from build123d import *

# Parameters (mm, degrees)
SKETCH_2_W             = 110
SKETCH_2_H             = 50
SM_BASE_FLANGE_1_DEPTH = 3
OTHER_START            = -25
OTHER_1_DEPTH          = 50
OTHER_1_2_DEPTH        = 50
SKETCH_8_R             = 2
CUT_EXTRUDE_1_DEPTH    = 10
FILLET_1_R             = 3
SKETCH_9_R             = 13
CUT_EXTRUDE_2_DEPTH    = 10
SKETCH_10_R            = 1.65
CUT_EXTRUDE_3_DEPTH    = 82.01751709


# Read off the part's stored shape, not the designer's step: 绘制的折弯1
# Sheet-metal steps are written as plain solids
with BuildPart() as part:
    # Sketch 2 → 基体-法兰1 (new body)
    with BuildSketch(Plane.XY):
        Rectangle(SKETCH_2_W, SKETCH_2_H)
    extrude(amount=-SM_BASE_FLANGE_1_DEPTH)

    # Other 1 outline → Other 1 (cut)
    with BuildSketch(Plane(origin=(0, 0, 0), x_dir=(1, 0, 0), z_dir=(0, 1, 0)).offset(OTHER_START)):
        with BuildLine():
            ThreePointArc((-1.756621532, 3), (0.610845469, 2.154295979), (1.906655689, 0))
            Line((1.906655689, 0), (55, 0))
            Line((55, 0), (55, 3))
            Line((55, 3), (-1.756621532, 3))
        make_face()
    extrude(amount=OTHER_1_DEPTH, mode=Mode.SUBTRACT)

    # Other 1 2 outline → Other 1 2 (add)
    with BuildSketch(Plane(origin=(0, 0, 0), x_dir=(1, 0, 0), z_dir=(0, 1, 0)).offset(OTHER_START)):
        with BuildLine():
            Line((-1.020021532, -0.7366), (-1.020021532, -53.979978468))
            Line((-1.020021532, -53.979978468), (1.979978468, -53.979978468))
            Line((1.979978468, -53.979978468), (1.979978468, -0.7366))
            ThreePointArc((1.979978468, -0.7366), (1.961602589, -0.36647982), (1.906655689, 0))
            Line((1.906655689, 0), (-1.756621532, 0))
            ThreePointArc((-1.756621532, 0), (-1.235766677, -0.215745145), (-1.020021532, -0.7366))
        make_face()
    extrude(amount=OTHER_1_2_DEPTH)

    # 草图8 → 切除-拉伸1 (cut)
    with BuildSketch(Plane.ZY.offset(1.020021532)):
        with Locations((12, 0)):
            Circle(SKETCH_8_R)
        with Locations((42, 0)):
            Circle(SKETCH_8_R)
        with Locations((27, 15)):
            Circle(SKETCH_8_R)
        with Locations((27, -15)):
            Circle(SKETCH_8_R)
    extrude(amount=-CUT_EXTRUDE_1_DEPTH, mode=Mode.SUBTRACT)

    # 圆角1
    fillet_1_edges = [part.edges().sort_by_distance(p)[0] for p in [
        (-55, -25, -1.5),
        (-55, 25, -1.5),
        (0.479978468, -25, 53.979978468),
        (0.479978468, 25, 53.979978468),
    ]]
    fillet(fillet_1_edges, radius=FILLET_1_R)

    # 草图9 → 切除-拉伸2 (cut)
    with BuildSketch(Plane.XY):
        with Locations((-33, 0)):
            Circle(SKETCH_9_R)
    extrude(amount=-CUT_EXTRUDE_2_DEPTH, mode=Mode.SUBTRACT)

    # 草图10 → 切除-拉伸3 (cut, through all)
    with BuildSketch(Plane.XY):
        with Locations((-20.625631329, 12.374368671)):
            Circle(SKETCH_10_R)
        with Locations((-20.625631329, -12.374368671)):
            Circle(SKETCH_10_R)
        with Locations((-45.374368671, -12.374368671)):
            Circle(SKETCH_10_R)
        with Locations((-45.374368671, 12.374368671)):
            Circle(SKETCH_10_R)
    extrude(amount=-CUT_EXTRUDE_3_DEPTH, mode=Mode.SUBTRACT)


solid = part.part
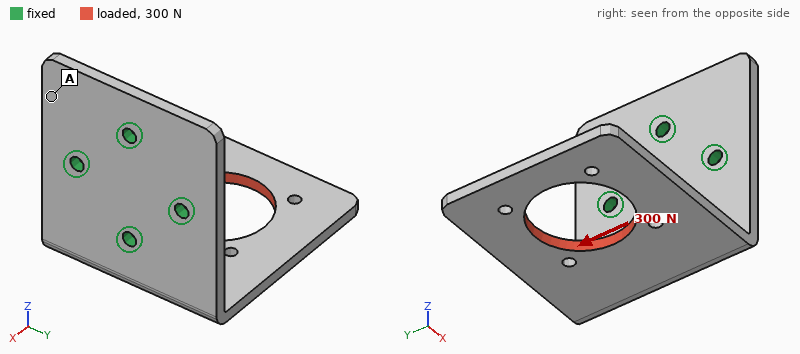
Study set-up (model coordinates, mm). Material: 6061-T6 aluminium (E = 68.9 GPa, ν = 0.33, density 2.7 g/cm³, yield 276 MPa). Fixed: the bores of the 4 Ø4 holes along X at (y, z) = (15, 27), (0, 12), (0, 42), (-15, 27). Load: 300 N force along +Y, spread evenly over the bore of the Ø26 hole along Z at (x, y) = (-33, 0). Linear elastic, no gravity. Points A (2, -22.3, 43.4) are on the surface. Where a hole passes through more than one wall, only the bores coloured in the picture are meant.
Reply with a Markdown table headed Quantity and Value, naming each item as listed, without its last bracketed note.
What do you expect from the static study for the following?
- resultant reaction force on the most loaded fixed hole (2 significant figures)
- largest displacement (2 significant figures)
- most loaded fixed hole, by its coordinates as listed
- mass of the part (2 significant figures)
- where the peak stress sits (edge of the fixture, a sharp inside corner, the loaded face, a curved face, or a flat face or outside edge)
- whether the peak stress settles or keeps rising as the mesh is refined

| Quantity | Value |
|---|---|
| resultant reaction force on the most loaded fixed hole | 280 N |
| largest displacement | 0.57 mm |
| most loaded fixed hole, by its coordinates as listed | (0, 12) |
| mass of the part | 40 g |
| where the peak stress sits | edge of the fixture |
| whether the peak stress settles or keeps rising as the mesh is refined | keeps rising |
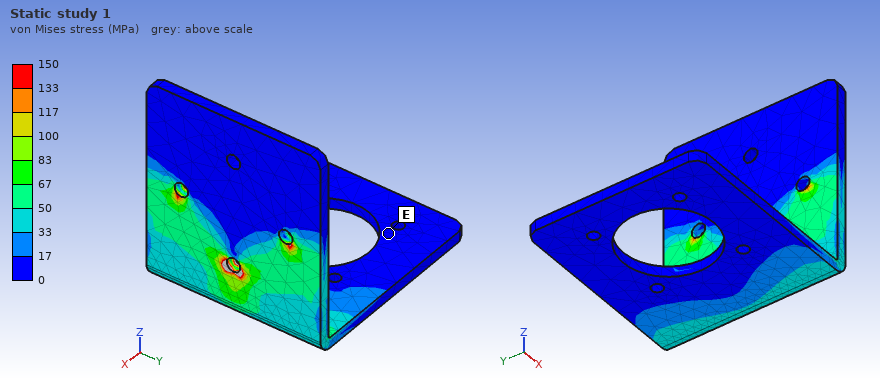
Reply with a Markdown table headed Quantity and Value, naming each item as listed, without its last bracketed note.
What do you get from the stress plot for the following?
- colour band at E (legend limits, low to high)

| Quantity | Value |
|---|---|
| colour band at E | 0 to 17 MPa |
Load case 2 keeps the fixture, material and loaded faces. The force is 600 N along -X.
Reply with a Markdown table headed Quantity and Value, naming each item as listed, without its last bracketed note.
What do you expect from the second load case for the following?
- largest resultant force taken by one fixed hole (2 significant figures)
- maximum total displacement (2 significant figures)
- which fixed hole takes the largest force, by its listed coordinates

| Quantity | Value |
|---|---|
| largest resultant force taken by one fixed hole | 760 N |
| maximum total displacement | 0.50 mm |
| which fixed hole takes the largest force, by its listed coordinates | (0, 12) |
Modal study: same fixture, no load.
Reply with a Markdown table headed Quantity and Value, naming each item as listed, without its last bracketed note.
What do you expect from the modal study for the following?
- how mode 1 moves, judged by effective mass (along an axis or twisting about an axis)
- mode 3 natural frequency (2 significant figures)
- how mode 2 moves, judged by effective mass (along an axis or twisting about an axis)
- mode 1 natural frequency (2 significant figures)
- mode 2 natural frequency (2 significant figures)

| Quantity | Value |
|---|---|
| how mode 1 moves, judged by effective mass | along Z |
| mode 3 natural frequency | 1800 Hz |
| how mode 2 moves, judged by effective mass | along Y |
| mode 1 natural frequency | 620 Hz |
| mode 2 natural frequency | 1100 Hz |
